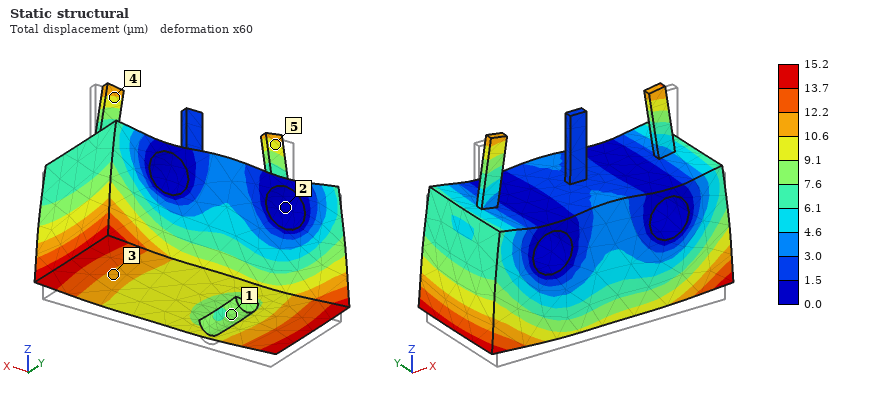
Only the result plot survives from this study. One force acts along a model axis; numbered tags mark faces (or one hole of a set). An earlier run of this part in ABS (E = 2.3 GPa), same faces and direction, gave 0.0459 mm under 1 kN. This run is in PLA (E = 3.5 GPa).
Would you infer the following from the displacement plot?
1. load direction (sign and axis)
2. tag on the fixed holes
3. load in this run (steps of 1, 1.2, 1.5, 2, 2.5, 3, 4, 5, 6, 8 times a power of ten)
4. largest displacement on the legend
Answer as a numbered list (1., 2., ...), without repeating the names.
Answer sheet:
1. +Z
2. 2
3. 500 N
4. 15.2 µm
